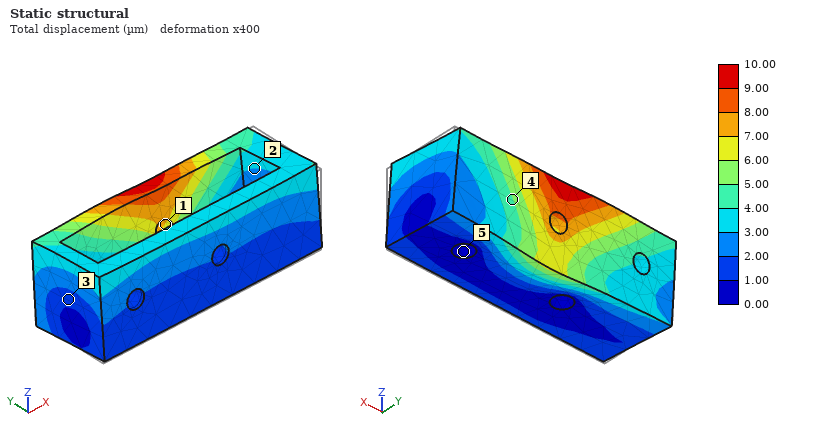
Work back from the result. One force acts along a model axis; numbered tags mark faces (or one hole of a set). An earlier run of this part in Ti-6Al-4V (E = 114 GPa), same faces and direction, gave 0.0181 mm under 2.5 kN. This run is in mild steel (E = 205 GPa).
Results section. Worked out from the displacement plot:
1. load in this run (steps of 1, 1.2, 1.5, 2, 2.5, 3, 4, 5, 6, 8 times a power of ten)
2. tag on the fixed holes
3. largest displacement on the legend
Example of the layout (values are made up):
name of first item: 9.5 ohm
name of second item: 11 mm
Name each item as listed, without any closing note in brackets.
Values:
load in this run: 2.5 kN
tag on the fixed holes: 5
largest displacement on the legend: 10.00 µm
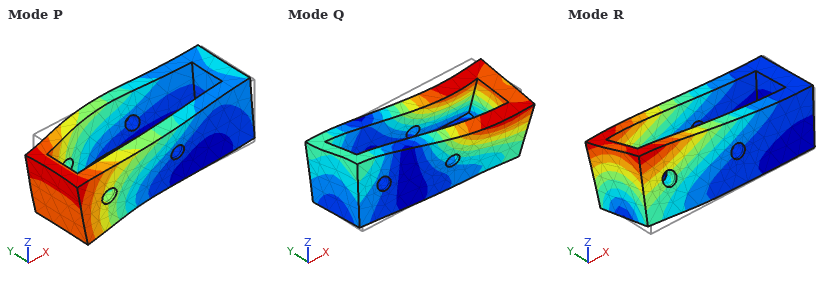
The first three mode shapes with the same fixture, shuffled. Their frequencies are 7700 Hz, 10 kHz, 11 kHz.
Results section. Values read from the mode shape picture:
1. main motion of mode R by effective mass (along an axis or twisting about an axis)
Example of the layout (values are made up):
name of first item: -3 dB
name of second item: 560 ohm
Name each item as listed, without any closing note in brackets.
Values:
main motion of mode R by effective mass: along Y
